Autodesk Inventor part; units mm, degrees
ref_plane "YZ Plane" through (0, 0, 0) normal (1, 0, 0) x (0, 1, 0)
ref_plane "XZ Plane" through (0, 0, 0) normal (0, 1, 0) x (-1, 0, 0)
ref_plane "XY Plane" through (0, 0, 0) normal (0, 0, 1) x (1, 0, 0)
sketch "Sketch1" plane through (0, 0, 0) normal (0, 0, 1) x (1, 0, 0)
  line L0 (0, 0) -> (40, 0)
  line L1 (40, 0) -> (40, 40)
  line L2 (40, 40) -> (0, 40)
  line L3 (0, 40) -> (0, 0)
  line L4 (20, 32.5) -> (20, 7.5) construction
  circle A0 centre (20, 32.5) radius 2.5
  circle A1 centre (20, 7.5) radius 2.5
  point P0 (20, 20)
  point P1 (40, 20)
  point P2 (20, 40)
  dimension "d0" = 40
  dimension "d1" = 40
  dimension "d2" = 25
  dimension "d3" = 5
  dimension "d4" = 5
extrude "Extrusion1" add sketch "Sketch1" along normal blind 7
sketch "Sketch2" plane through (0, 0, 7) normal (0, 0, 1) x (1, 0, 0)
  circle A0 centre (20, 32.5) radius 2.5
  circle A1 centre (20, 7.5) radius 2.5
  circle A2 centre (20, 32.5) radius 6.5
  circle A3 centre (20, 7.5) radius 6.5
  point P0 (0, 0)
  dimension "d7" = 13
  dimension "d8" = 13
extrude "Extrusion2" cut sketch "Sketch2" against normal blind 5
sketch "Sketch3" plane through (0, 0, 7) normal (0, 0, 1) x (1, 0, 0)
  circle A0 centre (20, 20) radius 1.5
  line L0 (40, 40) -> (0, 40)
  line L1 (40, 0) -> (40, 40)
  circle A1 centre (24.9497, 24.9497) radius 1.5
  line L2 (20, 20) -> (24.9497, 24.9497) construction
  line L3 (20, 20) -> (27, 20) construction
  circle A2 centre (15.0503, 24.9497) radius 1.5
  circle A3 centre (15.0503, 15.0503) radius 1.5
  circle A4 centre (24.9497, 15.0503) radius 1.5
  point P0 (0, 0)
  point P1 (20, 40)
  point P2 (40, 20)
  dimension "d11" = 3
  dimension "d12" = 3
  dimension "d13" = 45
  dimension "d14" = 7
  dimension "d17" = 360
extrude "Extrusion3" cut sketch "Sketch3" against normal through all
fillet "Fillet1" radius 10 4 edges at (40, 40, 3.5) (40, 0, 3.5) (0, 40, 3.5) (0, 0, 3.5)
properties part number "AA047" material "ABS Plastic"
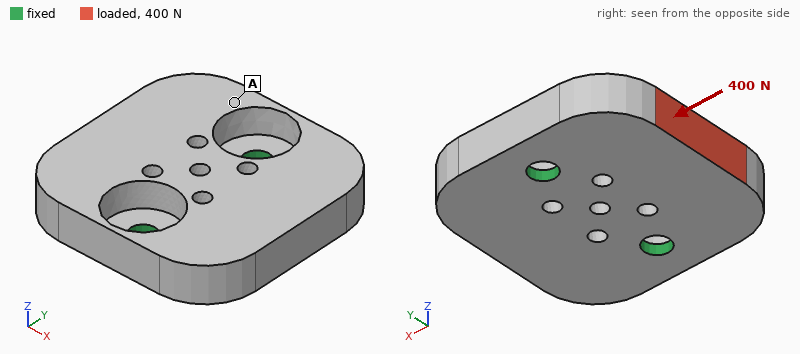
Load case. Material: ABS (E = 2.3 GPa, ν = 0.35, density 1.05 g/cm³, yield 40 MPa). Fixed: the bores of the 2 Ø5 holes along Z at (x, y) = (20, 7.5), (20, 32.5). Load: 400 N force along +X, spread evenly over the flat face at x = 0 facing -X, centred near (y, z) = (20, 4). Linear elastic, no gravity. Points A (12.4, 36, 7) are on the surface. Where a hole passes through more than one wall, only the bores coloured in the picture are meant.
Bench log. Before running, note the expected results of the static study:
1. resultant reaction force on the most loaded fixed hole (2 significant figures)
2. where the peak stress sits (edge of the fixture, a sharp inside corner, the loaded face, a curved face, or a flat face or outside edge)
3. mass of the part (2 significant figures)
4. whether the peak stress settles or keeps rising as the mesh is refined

200 N
edge of the fixture
9.4 g
keeps rising
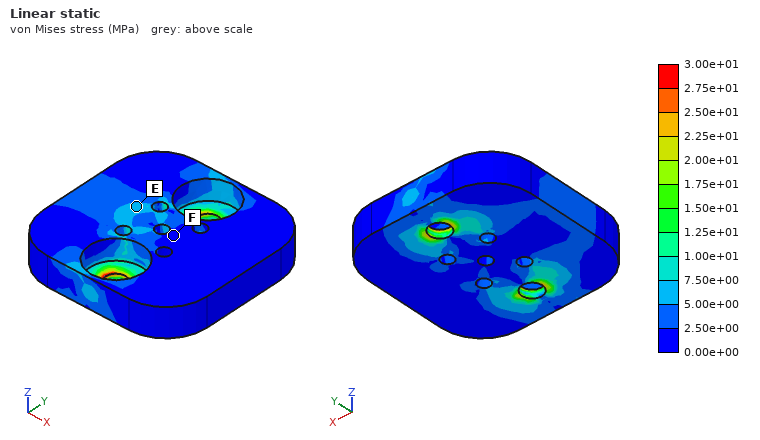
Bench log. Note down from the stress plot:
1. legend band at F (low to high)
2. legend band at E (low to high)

0.00e+00 to 2.50e+00 MPa
5.00e+00 to 7.50e+00 MPa
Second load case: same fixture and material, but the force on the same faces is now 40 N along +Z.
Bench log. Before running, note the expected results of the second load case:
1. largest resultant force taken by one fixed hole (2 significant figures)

25 N
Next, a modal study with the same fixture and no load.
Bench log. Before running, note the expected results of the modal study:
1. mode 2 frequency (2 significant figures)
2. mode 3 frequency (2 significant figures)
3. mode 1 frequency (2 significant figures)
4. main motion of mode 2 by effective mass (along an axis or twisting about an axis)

2700 Hz
3800 Hz
1100 Hz
along Z
